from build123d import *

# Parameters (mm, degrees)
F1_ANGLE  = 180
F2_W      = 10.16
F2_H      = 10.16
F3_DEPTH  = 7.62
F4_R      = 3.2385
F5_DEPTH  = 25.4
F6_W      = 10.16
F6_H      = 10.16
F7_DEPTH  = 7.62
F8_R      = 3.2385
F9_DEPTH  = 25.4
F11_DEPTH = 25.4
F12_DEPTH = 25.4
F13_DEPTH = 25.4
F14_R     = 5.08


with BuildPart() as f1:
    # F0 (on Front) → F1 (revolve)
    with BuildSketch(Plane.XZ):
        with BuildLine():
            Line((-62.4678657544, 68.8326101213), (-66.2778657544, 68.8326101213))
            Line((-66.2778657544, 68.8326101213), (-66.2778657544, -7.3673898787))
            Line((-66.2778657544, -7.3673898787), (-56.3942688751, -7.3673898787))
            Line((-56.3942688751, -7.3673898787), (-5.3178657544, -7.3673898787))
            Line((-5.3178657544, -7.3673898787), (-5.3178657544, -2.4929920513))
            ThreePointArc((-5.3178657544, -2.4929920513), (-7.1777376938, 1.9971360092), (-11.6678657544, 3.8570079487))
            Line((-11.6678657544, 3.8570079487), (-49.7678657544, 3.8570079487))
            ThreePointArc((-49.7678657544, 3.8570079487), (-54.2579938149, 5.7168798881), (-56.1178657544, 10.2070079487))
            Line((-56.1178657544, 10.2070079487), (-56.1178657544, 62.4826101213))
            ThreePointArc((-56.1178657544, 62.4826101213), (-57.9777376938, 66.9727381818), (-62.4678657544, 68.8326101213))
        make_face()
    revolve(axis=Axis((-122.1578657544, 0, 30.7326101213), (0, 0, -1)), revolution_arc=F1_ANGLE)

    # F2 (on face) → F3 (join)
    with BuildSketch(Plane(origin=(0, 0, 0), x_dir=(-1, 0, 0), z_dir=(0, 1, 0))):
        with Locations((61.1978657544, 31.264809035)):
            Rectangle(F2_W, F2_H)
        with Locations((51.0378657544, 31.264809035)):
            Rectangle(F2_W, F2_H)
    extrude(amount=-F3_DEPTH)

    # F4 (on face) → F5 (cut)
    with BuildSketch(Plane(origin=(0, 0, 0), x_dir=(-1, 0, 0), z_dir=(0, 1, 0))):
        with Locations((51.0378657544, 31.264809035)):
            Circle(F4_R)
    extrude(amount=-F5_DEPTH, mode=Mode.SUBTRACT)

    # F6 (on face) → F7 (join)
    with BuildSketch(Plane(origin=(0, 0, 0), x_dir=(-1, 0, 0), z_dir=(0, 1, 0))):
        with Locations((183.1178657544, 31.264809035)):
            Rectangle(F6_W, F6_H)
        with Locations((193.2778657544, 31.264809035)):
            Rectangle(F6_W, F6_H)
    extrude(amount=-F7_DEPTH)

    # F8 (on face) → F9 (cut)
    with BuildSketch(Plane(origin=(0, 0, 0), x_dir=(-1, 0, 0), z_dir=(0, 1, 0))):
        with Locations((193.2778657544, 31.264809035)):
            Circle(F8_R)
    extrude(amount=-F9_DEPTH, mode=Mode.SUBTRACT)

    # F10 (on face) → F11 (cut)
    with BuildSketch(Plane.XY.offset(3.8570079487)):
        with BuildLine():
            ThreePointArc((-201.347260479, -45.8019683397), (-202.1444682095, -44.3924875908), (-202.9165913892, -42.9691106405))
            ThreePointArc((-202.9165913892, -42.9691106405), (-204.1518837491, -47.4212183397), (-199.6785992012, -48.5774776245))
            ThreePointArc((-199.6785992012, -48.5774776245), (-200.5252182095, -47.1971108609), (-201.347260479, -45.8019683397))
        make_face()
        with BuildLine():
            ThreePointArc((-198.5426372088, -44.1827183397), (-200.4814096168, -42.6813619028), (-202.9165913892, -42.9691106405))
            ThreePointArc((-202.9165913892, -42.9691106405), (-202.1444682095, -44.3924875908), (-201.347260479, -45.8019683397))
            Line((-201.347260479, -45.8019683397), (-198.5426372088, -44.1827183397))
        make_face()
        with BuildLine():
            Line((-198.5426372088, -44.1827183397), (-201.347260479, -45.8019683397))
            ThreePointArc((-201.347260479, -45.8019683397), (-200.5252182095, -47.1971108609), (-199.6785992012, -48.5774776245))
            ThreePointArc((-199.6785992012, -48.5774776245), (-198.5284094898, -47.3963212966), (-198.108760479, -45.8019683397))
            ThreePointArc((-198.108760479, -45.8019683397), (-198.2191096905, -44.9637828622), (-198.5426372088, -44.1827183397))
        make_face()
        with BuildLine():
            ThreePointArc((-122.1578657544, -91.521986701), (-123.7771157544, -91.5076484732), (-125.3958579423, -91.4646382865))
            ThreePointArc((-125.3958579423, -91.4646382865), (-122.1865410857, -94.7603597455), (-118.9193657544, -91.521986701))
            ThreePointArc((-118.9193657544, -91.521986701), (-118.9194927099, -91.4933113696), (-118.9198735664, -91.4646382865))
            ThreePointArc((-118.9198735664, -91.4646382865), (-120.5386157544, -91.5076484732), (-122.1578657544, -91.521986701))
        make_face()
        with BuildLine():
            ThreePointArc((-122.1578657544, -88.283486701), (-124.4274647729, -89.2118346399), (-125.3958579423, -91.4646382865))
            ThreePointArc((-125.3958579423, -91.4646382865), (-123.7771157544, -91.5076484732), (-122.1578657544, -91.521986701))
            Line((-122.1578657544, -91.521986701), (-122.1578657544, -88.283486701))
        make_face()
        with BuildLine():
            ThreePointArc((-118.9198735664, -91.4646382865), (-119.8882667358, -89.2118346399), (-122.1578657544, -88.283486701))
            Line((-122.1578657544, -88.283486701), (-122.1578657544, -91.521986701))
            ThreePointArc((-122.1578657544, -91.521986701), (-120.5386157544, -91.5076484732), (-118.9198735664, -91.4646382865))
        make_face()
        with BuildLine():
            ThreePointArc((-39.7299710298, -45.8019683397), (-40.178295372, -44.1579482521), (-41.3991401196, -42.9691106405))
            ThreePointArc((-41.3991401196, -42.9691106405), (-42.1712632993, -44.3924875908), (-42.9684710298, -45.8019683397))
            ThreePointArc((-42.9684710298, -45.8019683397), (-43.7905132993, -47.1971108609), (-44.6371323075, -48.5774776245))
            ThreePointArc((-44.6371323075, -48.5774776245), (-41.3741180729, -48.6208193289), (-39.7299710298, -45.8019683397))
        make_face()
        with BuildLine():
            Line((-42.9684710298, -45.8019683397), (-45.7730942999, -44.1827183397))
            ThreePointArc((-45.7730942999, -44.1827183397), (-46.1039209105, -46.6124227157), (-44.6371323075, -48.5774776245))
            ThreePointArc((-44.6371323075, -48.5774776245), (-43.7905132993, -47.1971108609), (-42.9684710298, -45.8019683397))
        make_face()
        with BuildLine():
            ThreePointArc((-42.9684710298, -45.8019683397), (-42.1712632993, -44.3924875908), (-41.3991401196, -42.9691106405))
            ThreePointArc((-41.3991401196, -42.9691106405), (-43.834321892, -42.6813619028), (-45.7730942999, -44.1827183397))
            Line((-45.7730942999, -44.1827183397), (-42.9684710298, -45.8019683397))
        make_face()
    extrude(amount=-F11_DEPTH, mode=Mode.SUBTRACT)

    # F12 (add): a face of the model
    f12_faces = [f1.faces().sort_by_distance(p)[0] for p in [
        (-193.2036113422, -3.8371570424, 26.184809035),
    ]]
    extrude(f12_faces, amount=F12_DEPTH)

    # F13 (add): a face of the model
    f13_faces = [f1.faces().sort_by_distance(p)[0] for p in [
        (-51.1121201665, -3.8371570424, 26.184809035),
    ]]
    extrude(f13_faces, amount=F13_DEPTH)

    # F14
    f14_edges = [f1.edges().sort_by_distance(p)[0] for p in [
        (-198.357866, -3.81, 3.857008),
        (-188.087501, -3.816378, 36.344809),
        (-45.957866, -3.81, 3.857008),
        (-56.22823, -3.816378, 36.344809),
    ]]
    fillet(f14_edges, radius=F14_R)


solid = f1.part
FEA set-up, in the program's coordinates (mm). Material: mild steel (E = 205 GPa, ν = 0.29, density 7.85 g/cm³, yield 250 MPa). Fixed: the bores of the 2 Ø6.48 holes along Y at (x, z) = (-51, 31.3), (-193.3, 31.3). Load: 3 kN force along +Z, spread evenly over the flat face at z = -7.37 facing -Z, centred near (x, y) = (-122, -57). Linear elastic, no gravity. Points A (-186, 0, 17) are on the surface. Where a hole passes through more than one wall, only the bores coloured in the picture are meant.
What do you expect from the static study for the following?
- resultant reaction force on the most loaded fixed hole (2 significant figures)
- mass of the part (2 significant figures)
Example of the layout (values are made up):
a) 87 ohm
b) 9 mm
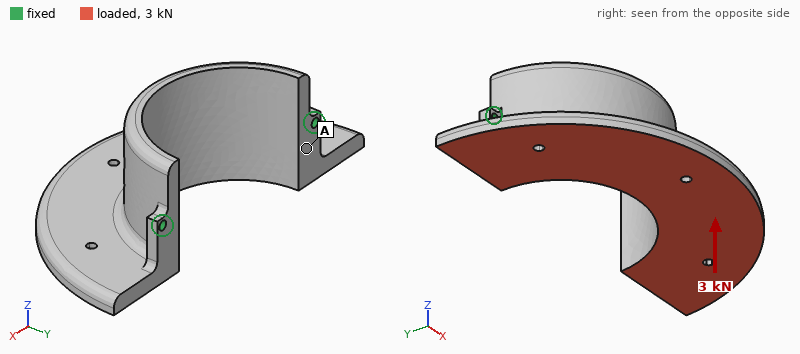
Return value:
a) 1.6 kN
b) 2.5 kg
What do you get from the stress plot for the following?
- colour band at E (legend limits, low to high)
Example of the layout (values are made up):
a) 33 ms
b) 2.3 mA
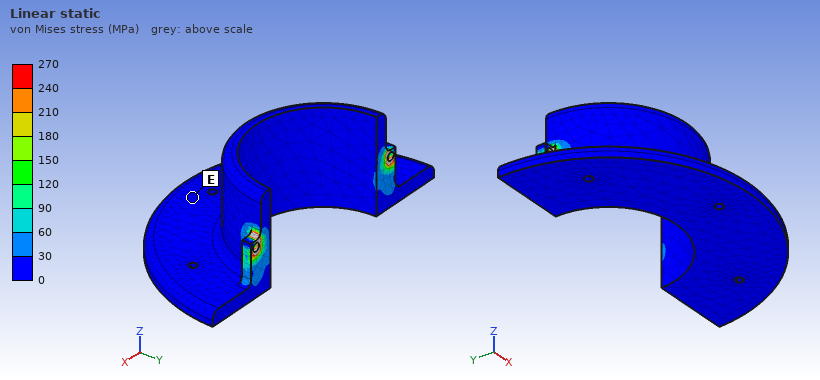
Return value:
a) 0 to 30 MPa
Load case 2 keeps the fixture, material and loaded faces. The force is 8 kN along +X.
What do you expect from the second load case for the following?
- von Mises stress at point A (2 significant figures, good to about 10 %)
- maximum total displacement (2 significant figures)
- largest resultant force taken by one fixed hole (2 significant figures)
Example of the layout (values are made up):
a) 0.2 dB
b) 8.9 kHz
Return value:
a) 29 MPa
b) 52 µm
c) 5.4 kN
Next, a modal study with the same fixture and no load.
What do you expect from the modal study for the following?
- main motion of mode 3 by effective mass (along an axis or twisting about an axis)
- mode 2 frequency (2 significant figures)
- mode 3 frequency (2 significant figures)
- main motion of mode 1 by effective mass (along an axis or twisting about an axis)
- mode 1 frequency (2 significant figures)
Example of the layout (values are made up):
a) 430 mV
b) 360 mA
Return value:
a) along X
b) 1200 Hz
c) 2100 Hz
d) along Z
e) 410 Hz
